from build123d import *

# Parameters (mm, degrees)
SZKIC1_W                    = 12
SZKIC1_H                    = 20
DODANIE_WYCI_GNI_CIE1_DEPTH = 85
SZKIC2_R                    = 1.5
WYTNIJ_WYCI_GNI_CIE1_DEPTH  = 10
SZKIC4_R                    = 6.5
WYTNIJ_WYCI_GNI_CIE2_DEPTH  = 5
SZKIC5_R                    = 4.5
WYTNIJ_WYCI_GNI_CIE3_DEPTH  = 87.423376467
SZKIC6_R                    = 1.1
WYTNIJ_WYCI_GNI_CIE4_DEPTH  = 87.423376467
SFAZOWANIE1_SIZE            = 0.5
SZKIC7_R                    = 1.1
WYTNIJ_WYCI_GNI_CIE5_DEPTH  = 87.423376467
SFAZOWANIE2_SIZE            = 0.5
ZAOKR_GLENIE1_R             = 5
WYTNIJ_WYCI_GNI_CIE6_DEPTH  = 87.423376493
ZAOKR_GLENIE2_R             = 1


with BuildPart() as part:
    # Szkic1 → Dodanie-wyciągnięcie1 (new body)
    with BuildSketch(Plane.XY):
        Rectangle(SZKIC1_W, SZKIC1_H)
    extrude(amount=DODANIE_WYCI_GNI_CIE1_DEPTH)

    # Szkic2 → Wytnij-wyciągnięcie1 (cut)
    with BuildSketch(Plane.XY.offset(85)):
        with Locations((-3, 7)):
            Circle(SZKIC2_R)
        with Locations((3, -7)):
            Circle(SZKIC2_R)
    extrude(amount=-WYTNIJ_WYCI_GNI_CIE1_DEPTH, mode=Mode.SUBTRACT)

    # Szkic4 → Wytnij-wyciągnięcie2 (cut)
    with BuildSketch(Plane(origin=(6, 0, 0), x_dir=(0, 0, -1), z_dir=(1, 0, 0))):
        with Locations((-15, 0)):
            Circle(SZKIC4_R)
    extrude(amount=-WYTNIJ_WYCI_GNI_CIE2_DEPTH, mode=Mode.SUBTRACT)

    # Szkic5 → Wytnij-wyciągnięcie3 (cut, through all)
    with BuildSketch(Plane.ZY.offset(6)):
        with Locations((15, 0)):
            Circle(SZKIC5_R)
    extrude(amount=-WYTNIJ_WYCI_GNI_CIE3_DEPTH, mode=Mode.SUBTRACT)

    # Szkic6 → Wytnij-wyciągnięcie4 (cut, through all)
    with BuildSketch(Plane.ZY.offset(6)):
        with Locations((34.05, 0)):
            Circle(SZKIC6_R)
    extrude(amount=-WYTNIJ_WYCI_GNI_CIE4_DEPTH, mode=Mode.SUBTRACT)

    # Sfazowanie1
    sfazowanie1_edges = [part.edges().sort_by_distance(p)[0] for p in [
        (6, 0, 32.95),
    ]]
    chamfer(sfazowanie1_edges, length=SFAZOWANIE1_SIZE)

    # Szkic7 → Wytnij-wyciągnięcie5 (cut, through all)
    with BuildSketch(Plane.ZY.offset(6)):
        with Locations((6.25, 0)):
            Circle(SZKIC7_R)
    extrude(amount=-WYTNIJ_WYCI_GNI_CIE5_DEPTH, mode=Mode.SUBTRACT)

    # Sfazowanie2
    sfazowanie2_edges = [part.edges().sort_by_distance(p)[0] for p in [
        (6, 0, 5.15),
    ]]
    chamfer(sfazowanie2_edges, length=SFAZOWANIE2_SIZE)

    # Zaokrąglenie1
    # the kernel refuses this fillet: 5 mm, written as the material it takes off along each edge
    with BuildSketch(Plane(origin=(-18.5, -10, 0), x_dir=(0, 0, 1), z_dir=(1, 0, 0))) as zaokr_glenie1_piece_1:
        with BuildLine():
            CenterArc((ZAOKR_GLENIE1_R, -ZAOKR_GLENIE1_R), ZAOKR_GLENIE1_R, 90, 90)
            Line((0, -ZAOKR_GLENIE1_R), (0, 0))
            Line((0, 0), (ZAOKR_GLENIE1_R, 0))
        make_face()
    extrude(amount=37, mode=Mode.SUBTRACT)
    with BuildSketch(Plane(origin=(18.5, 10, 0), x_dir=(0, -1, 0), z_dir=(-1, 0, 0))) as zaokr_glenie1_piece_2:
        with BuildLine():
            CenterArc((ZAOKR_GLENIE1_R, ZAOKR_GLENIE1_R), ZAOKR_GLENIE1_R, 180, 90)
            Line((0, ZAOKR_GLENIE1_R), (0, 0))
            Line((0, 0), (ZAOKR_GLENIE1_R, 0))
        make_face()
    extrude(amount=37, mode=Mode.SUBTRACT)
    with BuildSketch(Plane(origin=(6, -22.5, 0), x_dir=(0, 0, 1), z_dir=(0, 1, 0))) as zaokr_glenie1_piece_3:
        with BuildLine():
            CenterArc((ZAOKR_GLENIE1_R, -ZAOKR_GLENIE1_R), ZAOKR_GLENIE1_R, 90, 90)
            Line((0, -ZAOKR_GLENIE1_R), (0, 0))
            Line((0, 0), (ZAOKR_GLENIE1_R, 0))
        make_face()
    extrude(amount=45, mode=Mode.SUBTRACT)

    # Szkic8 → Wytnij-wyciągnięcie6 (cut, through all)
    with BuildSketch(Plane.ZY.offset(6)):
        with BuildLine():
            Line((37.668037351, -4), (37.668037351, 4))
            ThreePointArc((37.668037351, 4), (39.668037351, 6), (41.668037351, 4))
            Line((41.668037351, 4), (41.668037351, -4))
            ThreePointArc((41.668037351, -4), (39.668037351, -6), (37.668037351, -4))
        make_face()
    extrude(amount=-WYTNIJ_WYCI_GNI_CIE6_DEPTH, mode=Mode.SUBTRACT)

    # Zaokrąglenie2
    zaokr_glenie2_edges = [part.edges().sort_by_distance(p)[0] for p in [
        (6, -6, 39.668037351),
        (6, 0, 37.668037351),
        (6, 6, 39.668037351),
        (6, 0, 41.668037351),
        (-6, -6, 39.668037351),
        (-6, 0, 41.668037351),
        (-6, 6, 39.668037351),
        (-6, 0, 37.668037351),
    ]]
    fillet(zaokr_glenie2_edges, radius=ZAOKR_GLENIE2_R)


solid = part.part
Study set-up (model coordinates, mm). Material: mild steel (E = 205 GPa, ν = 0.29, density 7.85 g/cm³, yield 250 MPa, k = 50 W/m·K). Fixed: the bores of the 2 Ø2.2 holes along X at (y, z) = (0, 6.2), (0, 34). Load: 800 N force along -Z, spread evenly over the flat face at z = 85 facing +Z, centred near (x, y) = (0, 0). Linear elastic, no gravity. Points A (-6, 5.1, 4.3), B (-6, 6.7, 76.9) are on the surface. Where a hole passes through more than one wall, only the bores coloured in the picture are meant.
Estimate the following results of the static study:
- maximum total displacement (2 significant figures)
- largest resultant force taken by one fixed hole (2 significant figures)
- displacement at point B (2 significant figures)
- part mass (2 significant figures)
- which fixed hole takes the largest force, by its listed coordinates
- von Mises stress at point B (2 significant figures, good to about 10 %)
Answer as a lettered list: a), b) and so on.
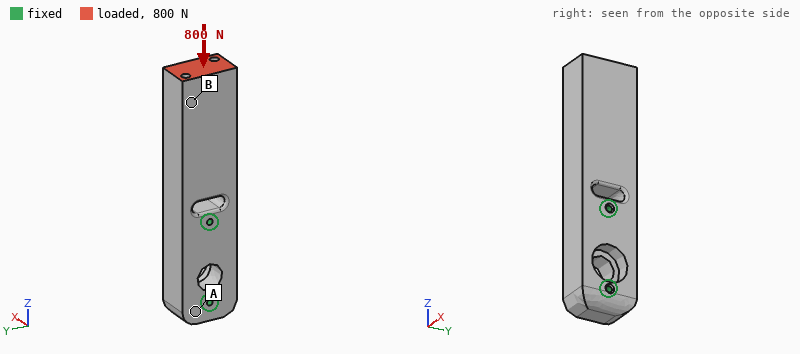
a) 1.5 µm
b) 640 N
c) 1.3 µm
d) 140 g
e) (0, 34)
f) 3.7 MPa
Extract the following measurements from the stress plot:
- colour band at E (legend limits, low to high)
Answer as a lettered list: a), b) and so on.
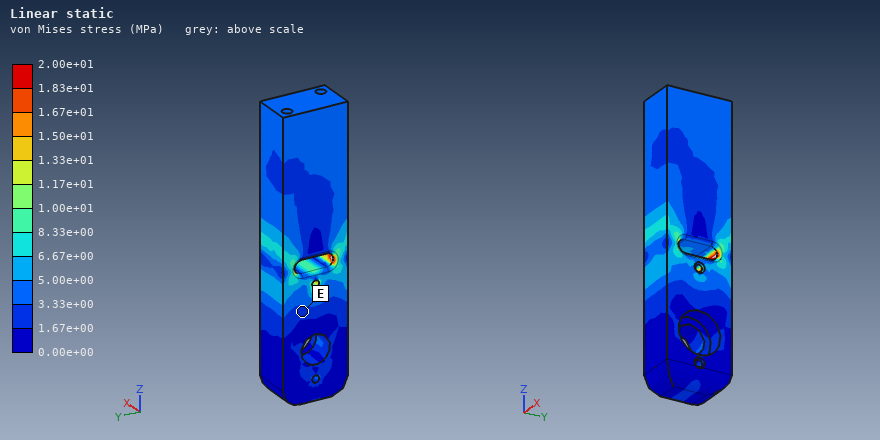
a) 1.67e+00 to 3.33e+00 MPa
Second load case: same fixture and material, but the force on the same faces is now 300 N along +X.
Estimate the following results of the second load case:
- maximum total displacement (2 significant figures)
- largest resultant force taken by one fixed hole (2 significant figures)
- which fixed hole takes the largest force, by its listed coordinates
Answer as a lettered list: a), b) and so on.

a) 51 µm
b) 620 N
c) (0, 34)
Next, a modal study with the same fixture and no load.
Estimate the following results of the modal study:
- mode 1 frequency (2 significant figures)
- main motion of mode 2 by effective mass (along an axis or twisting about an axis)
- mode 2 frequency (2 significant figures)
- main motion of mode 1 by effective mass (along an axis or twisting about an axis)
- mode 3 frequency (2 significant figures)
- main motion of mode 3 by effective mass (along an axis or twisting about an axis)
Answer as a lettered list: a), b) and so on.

a) 2400 Hz
b) along Y
c) 3800 Hz
d) along X
e) 10 kHz
f) twisting about Z
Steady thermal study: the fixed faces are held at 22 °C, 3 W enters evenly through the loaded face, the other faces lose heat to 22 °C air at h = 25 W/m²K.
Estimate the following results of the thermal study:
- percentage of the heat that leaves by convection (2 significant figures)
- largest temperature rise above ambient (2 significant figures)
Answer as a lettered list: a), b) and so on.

a) 26 %
b) 14 K
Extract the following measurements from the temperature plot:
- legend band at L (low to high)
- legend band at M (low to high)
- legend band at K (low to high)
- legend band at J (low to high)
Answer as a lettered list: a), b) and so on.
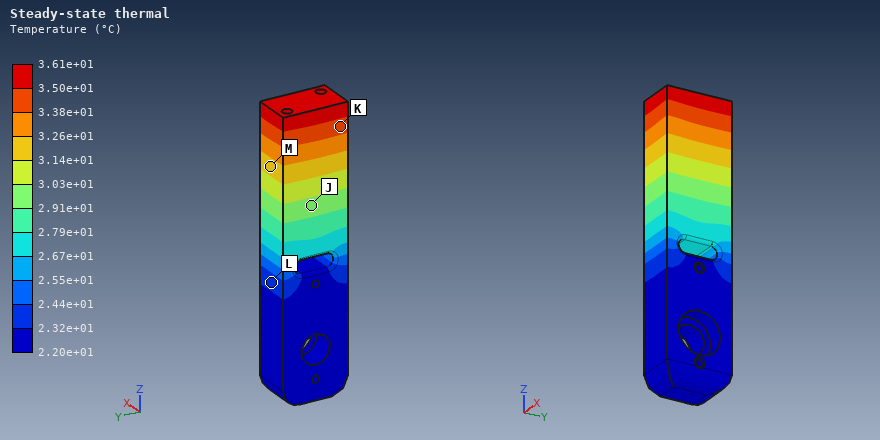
a) 2.32e+01 to 2.44e+01 °C
b) 3.14e+01 to 3.26e+01 °C
c) 3.38e+01 to 3.50e+01 °C
d) 2.91e+01 to 3.03e+01 °C
